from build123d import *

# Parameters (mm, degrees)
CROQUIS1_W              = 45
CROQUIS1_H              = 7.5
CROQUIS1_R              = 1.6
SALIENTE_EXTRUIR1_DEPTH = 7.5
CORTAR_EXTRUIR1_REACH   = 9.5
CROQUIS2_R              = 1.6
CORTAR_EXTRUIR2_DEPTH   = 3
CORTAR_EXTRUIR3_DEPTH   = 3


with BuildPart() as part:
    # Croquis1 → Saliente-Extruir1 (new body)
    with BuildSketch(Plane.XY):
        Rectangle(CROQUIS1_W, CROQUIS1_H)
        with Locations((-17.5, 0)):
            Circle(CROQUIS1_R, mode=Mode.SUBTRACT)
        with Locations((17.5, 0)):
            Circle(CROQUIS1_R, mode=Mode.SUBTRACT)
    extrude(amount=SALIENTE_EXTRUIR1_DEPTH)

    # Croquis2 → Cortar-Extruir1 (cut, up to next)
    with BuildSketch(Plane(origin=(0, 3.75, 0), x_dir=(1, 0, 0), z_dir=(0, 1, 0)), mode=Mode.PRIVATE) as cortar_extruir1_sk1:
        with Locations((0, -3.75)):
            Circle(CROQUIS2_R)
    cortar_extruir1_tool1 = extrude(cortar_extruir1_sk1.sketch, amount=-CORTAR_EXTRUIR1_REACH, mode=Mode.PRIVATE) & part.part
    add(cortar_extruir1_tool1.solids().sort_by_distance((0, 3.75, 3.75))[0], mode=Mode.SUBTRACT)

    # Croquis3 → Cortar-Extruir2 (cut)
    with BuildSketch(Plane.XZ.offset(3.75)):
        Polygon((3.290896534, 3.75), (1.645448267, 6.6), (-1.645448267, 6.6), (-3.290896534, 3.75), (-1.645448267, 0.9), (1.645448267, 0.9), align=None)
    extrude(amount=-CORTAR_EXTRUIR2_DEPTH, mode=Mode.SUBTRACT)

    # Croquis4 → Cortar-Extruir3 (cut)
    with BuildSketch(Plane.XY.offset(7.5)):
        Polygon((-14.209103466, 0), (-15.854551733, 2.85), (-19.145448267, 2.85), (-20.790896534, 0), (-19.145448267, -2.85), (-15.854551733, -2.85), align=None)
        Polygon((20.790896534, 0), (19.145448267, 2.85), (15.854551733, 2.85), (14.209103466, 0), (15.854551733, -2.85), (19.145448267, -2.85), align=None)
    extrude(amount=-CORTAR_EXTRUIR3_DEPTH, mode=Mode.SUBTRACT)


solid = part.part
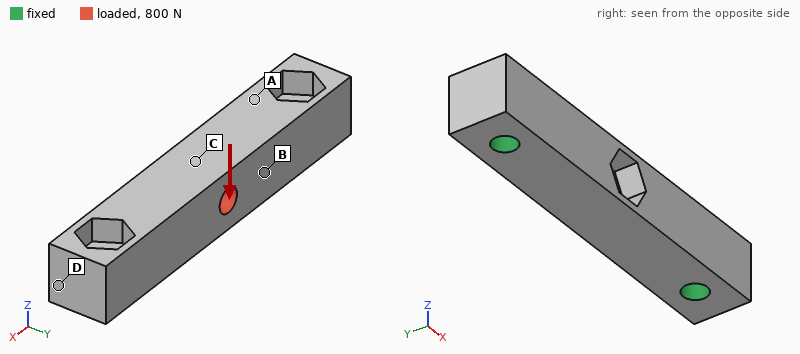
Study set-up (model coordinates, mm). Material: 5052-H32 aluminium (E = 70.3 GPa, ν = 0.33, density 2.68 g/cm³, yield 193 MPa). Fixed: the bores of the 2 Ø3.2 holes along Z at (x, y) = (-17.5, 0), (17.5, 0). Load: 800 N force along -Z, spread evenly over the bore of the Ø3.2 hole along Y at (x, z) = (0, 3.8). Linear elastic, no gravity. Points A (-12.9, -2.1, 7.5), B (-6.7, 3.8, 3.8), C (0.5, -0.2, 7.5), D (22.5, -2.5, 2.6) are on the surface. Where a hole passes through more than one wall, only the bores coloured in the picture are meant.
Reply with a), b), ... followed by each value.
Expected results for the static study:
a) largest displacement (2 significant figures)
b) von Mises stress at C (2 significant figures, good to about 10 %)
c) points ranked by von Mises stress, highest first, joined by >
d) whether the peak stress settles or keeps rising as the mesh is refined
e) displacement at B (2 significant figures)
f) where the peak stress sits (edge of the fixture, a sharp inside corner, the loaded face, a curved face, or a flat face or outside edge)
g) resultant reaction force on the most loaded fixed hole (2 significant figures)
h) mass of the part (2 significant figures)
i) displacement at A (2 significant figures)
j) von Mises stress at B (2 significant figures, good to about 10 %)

a) 24 µm
b) 76 MPa
c) C > B > A > D
d) keeps rising
e) 16 µm
f) edge of the fixture
g) 470 N
h) 5.8 g
i) 6.8 µm
j) 33 MPa
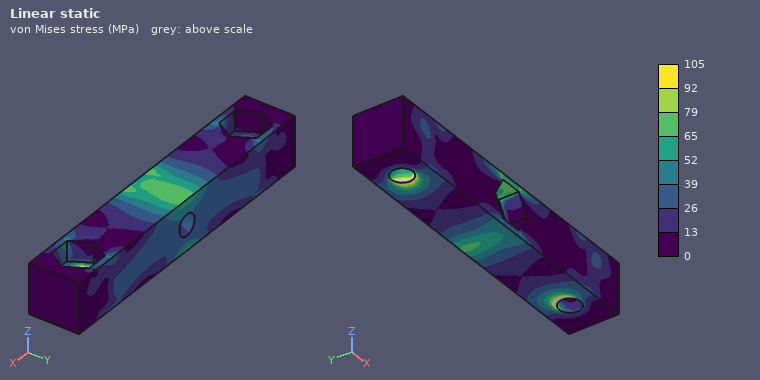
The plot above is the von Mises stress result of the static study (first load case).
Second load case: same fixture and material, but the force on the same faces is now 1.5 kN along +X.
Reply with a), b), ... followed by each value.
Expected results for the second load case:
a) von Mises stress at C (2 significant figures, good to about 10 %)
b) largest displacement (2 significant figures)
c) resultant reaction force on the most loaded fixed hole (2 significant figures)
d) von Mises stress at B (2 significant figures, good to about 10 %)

a) 7.2 MPa
b) 5.2 µm
c) 760 N
d) 23 MPa
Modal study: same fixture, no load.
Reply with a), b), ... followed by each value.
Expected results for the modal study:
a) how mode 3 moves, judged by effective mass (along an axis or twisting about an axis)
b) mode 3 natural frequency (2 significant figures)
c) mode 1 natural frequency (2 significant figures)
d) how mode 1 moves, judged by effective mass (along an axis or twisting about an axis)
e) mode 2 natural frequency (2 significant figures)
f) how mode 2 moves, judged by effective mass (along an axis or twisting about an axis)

a) twisting about X
b) 37 kHz
c) 20 kHz
d) along Y
e) 23 kHz
f) along Z
